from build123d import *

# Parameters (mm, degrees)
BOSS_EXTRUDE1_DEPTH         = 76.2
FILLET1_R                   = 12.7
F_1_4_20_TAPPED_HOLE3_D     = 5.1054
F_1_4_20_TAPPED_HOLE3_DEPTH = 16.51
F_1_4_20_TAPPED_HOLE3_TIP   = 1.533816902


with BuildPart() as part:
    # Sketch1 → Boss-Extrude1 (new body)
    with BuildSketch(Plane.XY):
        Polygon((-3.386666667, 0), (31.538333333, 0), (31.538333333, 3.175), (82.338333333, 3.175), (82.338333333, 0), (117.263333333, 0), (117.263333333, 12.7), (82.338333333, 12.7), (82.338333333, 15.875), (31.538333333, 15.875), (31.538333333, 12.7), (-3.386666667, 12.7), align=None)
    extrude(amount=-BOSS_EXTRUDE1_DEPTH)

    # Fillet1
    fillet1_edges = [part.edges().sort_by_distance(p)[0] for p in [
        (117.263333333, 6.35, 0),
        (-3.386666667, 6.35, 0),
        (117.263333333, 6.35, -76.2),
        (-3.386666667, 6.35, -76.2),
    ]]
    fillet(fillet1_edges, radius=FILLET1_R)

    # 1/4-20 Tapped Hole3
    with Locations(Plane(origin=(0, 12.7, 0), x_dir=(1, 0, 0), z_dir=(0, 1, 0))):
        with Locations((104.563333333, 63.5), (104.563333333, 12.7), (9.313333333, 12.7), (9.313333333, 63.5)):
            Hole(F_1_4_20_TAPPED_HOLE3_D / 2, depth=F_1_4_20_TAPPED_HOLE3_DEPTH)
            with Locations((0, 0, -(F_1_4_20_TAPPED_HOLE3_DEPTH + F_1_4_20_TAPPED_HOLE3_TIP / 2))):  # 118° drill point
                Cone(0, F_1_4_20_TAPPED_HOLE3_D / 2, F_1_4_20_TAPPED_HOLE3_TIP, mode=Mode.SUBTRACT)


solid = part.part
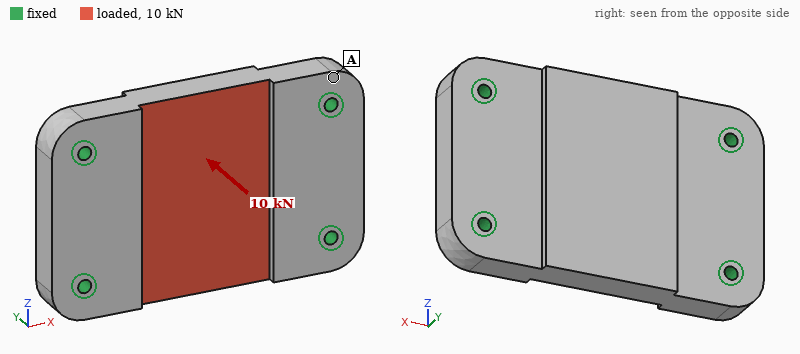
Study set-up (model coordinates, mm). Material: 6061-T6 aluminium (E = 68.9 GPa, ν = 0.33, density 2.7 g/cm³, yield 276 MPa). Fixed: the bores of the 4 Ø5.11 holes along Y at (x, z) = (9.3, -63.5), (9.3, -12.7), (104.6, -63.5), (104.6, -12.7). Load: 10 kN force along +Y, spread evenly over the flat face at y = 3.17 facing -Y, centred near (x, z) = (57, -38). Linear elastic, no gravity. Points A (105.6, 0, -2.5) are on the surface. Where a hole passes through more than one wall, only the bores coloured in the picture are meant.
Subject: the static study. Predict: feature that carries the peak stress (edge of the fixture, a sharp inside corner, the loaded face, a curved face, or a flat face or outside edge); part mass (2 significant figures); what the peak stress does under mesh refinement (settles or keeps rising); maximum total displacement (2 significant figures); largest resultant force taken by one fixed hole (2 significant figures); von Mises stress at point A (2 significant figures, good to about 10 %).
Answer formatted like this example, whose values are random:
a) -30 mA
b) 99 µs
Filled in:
a) edge of the fixture
b) 310 g
c) keeps rising
d) 59 µm
e) 3.4 kN
f) 22 MPa
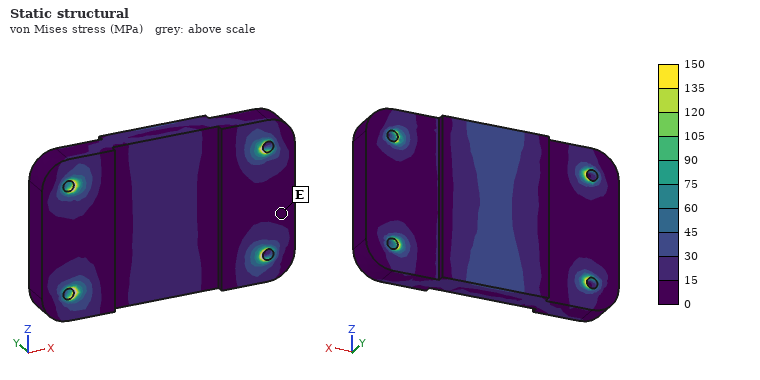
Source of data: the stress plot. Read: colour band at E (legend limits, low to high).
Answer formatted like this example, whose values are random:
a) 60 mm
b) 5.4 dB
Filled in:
a) 0 to 15 MPa
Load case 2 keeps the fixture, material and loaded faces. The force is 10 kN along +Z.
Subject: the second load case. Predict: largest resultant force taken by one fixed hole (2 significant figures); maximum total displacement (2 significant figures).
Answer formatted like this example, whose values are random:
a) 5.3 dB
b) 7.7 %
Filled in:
a) 2.9 kN
b) 17 µm
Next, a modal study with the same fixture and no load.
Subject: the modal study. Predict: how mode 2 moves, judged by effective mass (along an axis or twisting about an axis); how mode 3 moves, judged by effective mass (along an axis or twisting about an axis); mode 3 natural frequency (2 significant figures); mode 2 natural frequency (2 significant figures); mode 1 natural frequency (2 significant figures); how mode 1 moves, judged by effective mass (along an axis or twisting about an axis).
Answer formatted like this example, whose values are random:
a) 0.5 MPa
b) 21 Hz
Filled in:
a) twisting about X
b) along Z
c) 13 kHz
d) 7700 Hz
e) 5800 Hz
f) along Y
